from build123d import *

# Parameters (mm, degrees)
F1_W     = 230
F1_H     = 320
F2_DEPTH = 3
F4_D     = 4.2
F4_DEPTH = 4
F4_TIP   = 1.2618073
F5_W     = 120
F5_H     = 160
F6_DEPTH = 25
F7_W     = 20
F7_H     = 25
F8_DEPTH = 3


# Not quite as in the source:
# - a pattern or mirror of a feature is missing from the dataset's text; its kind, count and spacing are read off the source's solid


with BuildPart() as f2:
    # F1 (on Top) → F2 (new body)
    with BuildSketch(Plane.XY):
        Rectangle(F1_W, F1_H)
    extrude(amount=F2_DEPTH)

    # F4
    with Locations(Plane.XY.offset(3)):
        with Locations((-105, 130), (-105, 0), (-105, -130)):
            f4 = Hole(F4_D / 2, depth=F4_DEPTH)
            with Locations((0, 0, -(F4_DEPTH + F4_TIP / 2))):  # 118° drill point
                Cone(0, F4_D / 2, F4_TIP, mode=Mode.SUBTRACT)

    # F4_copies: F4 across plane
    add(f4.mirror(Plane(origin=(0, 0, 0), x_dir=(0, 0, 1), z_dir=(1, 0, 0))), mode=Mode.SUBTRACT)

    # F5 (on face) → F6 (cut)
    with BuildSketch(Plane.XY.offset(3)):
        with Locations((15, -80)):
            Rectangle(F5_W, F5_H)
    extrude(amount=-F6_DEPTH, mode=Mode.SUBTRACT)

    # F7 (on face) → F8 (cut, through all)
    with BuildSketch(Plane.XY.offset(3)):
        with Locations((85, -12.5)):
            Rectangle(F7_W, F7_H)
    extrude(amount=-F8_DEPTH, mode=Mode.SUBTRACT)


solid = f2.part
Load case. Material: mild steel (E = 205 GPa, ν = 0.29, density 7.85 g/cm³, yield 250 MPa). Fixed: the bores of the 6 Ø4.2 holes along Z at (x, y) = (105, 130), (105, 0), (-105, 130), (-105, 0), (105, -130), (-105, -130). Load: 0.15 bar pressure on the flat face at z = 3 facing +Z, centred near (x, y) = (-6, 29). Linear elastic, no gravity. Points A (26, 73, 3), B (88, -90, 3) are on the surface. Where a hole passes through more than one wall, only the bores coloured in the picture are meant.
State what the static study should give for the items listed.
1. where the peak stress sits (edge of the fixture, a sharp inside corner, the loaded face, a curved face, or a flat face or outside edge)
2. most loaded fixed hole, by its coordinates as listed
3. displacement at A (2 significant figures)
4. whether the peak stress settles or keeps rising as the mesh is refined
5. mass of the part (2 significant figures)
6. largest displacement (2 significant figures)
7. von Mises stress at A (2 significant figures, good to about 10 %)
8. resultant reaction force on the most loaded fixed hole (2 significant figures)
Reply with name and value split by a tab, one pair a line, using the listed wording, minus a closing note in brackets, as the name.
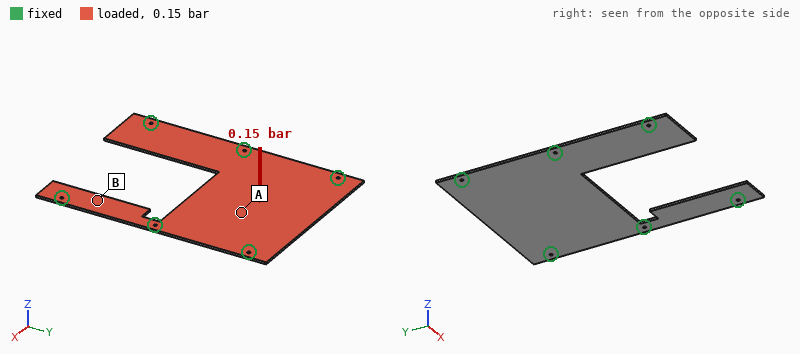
where the peak stress sits	edge of the fixture
most loaded fixed hole, by its coordinates as listed	(-105, 0)
displacement at A	0.25 mm
whether the peak stress settles or keeps rising as the mesh is refined	keeps rising
mass of the part	1.3 kg
largest displacement	0.27 mm
von Mises stress at A	17 MPa
resultant reaction force on the most loaded fixed hole	190 N
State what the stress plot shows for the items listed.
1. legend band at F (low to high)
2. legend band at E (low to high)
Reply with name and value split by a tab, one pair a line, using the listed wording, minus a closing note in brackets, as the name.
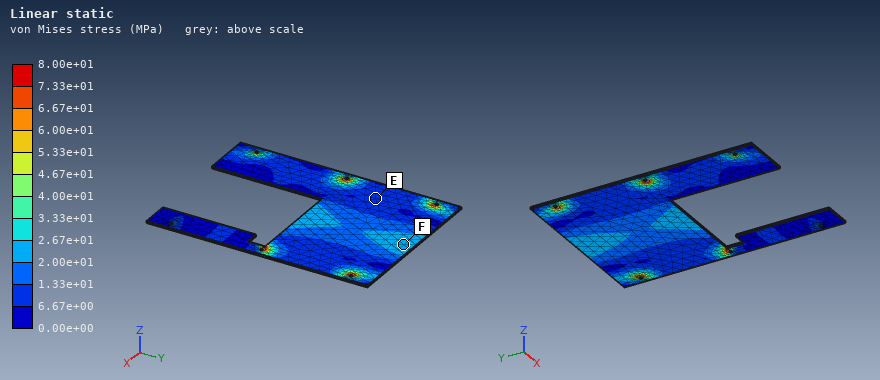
legend band at F	2.00e+01 to 2.67e+01 MPa
legend band at E	6.67e+00 to 1.33e+01 MPa
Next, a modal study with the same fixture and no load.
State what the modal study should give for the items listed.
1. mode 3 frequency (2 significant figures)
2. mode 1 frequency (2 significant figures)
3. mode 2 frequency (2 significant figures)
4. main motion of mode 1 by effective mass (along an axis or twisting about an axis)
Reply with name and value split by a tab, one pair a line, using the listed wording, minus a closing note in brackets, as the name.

mode 3 frequency	530 Hz
mode 1 frequency	290 Hz
mode 2 frequency	430 Hz
main motion of mode 1 by effective mass	along Z
